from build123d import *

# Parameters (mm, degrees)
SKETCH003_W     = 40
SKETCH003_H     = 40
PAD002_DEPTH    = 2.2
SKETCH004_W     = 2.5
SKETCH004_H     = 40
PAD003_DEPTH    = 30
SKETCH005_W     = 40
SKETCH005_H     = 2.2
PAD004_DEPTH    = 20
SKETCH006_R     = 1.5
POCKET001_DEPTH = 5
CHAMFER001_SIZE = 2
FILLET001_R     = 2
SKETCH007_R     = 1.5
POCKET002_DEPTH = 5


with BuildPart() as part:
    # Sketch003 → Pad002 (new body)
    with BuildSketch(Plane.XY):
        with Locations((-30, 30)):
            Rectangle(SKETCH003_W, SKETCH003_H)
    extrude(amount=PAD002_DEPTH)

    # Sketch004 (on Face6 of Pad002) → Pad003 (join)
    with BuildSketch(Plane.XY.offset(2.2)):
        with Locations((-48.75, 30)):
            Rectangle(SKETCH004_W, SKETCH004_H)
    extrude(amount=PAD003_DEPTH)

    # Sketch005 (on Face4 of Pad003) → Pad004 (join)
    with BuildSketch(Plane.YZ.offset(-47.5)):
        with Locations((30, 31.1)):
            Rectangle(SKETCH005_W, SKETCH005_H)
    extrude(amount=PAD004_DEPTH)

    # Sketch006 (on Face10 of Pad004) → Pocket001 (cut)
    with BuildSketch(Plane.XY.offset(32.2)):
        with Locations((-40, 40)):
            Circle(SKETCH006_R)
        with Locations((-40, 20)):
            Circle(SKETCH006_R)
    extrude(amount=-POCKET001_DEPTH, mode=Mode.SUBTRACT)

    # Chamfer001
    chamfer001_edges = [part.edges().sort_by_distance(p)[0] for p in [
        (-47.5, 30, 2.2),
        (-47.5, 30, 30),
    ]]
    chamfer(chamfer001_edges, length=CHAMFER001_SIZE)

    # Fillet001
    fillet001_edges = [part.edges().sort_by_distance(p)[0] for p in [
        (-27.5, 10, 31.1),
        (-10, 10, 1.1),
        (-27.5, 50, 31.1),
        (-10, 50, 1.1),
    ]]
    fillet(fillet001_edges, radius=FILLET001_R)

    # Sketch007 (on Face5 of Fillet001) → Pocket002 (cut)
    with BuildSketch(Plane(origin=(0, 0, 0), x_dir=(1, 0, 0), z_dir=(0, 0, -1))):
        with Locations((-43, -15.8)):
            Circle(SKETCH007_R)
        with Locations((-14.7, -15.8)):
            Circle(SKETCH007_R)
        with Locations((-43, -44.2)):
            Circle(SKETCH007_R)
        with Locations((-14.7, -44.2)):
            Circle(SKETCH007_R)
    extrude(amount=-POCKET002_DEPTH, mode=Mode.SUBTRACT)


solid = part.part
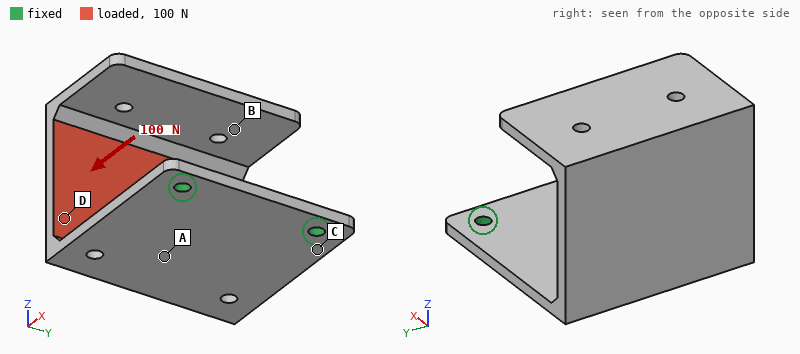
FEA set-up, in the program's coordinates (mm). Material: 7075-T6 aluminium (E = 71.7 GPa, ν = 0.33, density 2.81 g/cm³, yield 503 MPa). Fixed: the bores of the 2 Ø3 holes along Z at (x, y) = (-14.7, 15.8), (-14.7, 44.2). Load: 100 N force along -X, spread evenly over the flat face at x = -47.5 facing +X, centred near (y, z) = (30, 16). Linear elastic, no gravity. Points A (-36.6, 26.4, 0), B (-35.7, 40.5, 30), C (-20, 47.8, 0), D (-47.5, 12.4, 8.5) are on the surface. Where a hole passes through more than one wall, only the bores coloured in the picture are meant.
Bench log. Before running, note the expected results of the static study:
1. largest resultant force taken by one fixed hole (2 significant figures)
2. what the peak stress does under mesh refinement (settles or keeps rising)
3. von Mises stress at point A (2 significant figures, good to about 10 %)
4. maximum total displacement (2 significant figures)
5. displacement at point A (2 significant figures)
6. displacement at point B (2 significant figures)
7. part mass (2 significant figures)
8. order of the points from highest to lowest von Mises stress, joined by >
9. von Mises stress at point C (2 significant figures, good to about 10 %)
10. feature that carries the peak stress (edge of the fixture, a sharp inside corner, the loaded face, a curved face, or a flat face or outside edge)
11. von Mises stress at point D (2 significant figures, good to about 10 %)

51 N
keeps rising
41 MPa
0.76 mm
0.16 mm
0.61 mm
23 g
C > A > D > B
53 MPa
edge of the fixture
15 MPa
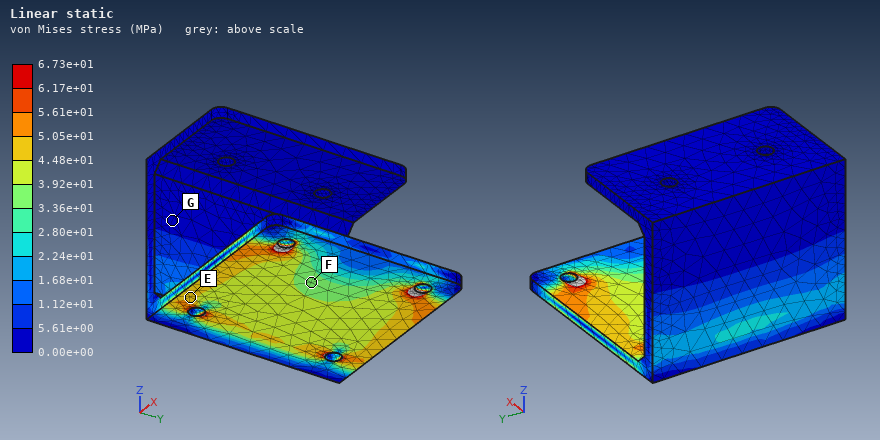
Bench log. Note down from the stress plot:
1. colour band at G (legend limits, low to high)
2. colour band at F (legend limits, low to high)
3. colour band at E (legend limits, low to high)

0.00e+00 to 5.61e+00 MPa
3.36e+01 to 3.92e+01 MPa
4.48e+01 to 5.05e+01 MPa
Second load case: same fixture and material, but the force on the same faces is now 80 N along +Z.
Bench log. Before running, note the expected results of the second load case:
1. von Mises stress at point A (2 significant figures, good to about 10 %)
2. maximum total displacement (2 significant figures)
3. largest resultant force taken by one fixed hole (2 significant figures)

25 MPa
0.70 mm
40 N
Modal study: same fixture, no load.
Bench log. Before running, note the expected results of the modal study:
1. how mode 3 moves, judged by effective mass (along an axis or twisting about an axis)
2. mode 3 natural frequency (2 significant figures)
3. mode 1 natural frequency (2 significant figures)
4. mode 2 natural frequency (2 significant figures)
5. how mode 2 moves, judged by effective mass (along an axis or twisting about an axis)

along Z
1000 Hz
400 Hz
710 Hz
along Y
